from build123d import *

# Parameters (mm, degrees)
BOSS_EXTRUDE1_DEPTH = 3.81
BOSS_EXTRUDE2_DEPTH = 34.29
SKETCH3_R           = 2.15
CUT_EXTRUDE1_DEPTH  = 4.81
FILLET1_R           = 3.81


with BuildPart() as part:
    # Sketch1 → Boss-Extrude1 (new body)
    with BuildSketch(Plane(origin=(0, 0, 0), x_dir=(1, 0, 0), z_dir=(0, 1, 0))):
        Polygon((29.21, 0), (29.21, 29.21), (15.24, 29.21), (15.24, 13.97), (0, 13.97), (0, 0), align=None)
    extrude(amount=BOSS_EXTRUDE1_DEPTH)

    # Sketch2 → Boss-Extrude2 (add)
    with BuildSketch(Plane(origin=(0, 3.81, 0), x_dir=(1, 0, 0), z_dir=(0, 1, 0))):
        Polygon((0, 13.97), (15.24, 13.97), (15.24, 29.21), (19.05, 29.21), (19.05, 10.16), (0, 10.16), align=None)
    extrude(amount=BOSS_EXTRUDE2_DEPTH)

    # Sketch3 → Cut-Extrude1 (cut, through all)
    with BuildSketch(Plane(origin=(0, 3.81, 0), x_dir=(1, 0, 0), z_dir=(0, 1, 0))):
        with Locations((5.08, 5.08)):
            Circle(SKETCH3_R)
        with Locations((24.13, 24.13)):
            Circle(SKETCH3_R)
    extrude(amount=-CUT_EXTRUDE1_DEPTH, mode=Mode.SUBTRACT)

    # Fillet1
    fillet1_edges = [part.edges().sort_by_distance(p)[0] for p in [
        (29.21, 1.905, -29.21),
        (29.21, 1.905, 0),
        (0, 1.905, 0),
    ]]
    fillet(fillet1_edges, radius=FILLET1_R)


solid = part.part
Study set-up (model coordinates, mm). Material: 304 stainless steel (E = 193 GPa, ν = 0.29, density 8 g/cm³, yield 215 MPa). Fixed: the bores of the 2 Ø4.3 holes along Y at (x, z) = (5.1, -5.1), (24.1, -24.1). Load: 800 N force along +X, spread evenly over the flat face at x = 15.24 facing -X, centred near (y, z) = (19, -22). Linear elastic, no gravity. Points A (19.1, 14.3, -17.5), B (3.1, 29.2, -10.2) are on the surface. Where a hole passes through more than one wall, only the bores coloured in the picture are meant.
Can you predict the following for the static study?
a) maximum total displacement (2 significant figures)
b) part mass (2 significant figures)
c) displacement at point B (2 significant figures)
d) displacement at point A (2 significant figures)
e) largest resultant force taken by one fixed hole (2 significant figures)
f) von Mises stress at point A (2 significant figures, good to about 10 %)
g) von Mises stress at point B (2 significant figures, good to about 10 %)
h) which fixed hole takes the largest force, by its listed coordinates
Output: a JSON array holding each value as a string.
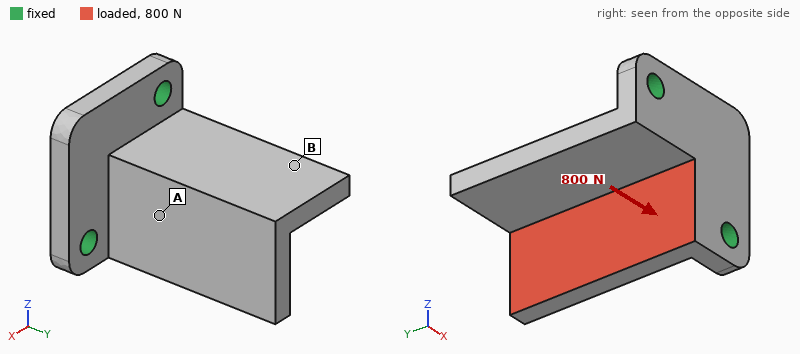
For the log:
["86 µm", "54 g", "28 µm", "21 µm", "670 N", "45 MPa", "13 MPa", "(24.1, -24.1)"]
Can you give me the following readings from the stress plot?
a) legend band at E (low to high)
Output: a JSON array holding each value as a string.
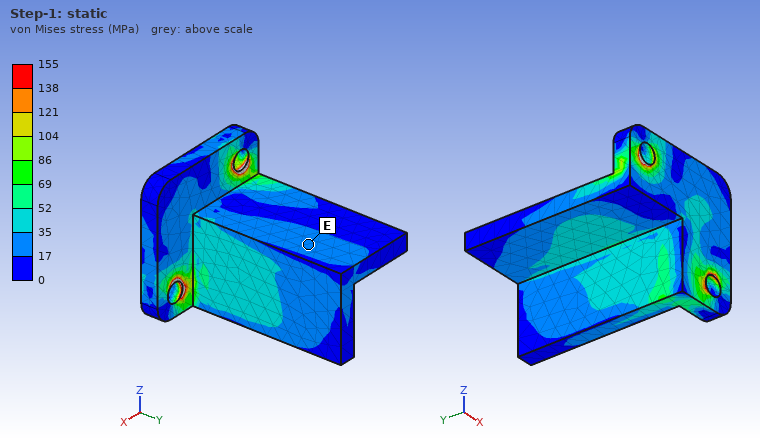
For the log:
["17 to 35 MPa"]
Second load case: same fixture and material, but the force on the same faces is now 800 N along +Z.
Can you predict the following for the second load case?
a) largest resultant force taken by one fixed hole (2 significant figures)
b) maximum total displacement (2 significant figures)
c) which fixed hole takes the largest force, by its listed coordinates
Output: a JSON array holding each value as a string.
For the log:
["720 N", "54 µm", "(24.1, -24.1)"]
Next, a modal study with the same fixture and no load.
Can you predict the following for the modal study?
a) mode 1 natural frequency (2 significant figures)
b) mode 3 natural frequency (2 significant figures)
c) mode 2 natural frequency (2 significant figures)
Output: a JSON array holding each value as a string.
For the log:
["3100 Hz", "7500 Hz", "5500 Hz"]
